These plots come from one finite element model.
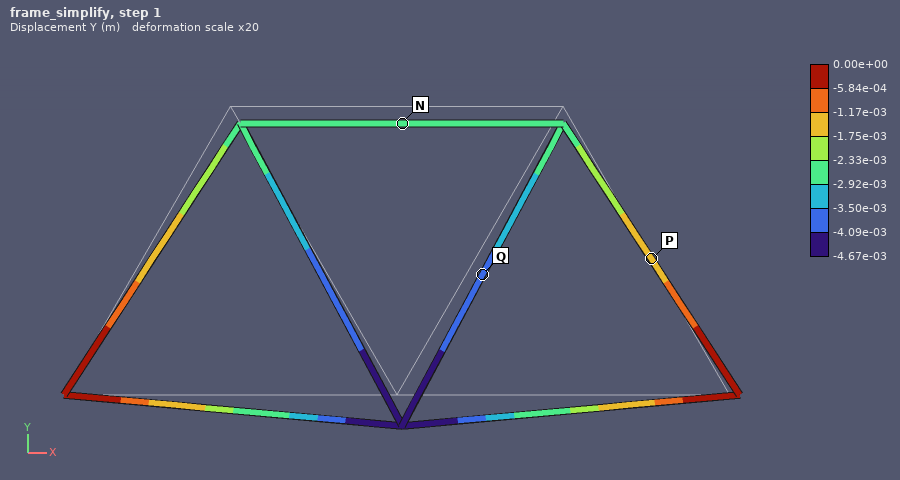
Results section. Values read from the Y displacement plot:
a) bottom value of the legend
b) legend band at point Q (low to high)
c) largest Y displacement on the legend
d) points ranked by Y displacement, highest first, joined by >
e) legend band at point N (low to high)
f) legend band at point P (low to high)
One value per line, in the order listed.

-4.67e-03 m
-4.09e-03 to -3.50e-03 m
0.00e+00 m
P > N > Q
-2.92e-03 to -2.33e-03 m
-1.75e-03 to -1.17e-03 m
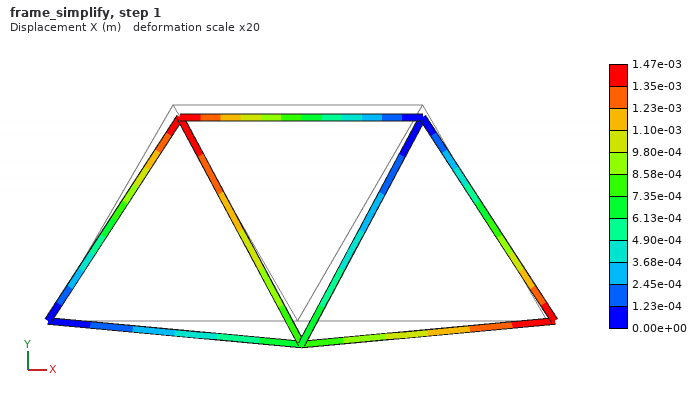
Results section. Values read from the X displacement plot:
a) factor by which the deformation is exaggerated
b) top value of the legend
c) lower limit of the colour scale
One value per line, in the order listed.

20
1.47e-03 m
0.00e+00 m
